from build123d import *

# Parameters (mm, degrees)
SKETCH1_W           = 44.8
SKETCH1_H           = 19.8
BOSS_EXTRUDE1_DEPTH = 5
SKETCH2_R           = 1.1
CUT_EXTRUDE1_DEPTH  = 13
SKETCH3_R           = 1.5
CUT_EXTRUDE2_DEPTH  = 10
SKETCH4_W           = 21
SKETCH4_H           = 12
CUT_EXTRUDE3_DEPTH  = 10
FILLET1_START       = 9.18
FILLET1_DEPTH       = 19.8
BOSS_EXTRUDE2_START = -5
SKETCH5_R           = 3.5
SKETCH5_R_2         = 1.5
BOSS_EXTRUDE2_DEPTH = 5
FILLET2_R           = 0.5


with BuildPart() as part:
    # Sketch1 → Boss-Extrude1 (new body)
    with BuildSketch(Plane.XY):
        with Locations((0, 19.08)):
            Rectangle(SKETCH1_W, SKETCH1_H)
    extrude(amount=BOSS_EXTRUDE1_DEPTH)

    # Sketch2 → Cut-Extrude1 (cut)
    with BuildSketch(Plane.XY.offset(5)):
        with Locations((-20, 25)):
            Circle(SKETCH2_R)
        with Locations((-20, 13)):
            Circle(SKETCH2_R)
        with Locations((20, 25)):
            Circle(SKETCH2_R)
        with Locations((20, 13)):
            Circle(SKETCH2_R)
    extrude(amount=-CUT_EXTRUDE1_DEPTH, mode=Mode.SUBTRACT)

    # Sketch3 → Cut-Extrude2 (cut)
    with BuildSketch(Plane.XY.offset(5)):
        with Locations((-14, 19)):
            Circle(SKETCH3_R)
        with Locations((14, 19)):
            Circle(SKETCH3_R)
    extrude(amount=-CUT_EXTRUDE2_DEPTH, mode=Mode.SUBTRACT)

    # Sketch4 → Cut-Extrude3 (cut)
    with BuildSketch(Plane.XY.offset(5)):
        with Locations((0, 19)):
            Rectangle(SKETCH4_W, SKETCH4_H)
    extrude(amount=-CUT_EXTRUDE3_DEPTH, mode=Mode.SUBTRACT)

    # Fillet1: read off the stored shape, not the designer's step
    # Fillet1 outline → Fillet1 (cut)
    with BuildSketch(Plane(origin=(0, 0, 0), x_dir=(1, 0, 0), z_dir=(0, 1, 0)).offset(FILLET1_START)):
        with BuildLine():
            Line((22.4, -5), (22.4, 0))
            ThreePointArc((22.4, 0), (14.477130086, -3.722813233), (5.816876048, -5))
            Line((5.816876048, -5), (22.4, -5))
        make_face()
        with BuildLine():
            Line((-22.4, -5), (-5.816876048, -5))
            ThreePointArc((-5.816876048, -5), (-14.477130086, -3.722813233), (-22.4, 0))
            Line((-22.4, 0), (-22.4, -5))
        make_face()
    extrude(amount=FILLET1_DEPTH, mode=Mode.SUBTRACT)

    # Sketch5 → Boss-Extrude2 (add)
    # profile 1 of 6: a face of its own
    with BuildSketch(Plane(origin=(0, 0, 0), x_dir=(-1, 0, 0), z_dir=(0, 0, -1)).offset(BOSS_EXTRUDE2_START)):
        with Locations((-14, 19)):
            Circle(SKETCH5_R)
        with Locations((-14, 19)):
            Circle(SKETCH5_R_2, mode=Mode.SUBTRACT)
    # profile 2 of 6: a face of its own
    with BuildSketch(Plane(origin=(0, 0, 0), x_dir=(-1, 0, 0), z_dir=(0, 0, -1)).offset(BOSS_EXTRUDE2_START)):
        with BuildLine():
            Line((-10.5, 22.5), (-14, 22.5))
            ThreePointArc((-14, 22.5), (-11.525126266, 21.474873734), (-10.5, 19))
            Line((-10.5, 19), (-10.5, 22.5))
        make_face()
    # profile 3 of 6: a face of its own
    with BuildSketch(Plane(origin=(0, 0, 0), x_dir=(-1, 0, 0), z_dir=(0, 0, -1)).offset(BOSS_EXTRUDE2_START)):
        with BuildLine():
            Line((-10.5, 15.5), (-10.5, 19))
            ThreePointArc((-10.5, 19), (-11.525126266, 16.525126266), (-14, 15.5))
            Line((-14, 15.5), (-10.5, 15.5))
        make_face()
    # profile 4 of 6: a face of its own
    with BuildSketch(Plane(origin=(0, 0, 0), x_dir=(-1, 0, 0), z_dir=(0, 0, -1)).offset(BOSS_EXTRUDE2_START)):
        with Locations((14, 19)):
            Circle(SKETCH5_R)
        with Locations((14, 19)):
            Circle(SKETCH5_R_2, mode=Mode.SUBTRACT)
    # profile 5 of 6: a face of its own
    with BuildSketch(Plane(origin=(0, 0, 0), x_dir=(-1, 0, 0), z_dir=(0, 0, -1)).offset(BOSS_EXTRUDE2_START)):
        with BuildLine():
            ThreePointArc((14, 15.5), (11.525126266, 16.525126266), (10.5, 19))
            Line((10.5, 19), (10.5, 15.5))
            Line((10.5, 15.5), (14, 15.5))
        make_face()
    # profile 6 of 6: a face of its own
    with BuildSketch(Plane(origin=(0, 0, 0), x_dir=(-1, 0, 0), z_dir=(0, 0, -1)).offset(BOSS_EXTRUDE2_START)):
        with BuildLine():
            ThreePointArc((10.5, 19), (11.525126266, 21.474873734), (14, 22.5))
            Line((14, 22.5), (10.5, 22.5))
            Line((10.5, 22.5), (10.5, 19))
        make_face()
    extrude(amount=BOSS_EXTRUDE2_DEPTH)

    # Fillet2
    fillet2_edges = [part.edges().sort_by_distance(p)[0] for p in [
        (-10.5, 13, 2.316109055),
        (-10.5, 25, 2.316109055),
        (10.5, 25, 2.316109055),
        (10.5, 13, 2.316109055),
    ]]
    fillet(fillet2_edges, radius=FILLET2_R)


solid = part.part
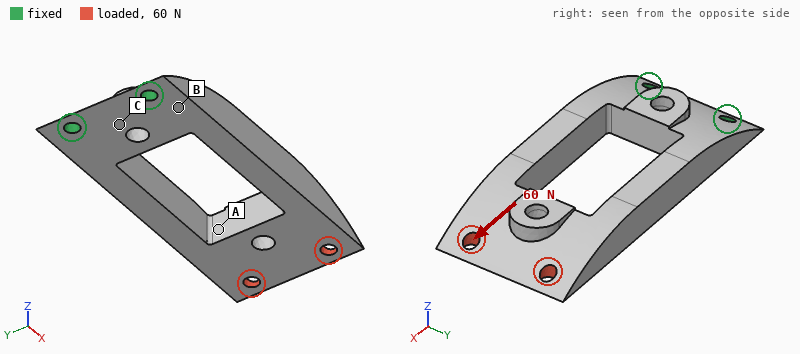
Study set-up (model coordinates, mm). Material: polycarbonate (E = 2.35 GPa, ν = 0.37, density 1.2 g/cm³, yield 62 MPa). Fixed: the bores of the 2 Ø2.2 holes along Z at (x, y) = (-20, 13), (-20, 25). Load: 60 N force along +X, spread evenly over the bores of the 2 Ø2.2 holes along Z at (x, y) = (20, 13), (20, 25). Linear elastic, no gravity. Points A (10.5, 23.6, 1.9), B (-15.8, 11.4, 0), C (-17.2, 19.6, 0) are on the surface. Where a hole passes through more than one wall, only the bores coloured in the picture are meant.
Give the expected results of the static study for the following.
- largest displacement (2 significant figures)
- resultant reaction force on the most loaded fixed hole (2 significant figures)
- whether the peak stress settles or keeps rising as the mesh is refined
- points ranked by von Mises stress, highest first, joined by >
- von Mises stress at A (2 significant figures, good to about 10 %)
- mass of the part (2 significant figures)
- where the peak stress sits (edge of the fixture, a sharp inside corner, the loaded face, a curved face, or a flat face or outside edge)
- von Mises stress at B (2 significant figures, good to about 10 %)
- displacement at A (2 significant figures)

0.50 mm
30 N
keeps rising
B > A > C
2.1 MPa
2.6 g
a sharp inside corner
4.0 MPa
0.25 mm
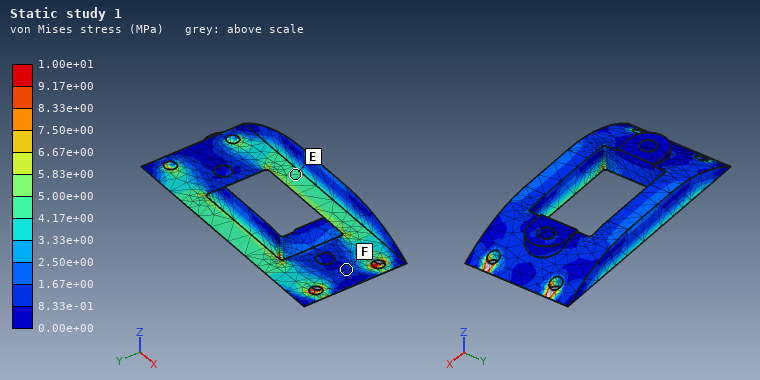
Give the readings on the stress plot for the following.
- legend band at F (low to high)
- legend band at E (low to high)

8.33e-01 to 1.67e+00 MPa
4.17e+00 to 5.00e+00 MPa
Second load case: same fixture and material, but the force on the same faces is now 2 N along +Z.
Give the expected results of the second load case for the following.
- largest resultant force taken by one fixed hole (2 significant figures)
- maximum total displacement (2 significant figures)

1.0 N
0.54 mm
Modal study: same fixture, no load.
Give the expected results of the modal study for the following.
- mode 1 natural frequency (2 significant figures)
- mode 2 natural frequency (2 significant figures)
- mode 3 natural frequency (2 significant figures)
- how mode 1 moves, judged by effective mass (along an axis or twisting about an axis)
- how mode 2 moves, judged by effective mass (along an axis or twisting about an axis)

360 Hz
1100 Hz
1500 Hz
along Z
along Y
